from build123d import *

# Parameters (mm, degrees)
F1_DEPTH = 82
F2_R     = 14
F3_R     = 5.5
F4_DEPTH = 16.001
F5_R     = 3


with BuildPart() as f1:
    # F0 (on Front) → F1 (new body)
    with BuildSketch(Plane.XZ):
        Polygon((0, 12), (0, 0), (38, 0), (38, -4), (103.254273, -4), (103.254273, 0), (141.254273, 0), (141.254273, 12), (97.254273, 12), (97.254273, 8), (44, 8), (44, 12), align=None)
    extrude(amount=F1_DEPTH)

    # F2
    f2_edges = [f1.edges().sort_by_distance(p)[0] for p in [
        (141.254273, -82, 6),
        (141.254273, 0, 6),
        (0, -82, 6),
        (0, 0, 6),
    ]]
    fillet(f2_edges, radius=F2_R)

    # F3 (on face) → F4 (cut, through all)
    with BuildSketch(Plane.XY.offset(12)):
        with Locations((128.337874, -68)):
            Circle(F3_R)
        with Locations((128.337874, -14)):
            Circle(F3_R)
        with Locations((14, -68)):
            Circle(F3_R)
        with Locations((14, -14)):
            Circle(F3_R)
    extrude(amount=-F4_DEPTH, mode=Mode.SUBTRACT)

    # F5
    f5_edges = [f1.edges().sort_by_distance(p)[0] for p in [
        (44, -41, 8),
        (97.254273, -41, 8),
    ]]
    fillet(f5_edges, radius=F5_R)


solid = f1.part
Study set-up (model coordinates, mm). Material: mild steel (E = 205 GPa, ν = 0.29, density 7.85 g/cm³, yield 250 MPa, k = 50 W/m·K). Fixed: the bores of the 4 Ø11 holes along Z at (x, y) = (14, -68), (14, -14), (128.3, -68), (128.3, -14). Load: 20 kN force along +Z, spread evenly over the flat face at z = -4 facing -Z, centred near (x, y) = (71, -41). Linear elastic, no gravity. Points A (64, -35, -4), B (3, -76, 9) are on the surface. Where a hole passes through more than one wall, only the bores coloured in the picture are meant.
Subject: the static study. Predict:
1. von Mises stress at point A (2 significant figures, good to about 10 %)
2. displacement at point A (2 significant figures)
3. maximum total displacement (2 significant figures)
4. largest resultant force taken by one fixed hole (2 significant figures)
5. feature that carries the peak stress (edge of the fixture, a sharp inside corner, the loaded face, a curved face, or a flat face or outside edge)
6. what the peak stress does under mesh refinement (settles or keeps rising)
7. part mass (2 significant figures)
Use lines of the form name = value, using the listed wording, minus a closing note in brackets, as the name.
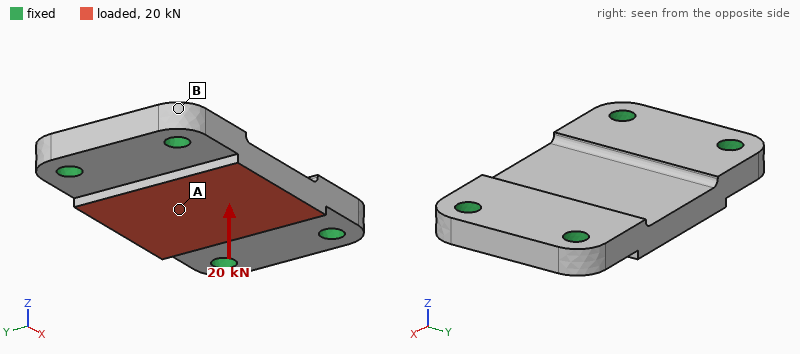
von Mises stress at point A = 62 MPa
displacement at point A = 42 µm
maximum total displacement = 45 µm
largest resultant force taken by one fixed hole = 8.3 kN
feature that carries the peak stress = edge of the fixture
what the peak stress does under mesh refinement = keeps rising
part mass = 1.1 kg
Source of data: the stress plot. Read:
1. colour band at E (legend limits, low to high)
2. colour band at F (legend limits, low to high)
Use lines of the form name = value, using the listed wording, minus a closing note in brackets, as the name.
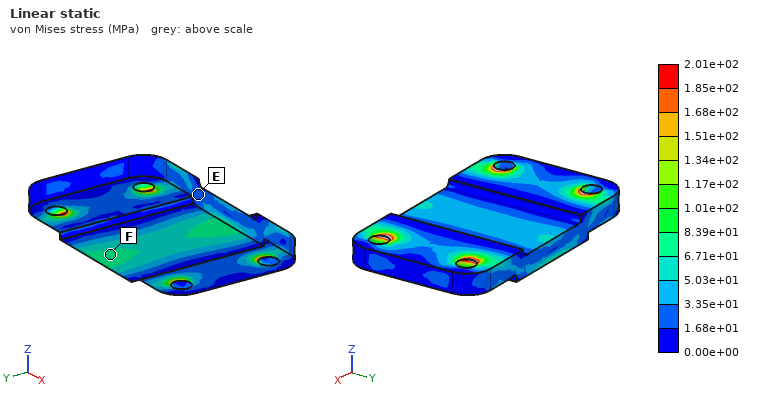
colour band at E = 1.68e+01 to 3.35e+01 MPa
colour band at F = 6.71e+01 to 8.39e+01 MPa
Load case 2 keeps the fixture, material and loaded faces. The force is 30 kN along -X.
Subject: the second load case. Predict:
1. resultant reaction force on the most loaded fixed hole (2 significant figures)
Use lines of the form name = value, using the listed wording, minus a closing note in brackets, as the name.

resultant reaction force on the most loaded fixed hole = 7.8 kN
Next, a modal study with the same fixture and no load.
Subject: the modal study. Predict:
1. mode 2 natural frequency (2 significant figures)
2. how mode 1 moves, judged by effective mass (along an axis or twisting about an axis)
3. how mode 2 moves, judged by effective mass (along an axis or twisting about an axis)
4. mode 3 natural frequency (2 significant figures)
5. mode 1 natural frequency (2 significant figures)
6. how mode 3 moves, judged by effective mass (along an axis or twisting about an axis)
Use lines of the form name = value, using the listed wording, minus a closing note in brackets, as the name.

mode 2 natural frequency = 6600 Hz
how mode 1 moves, judged by effective mass = along Z
how mode 2 moves, judged by effective mass = twisting about X
mode 3 natural frequency = 11 kHz
mode 1 natural frequency = 4900 Hz
how mode 3 moves, judged by effective mass = twisting about Y
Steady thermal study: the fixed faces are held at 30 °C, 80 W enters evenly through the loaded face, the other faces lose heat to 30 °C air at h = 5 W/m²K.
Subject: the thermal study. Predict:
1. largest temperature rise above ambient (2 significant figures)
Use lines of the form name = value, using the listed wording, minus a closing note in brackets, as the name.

largest temperature rise above ambient = 35 K
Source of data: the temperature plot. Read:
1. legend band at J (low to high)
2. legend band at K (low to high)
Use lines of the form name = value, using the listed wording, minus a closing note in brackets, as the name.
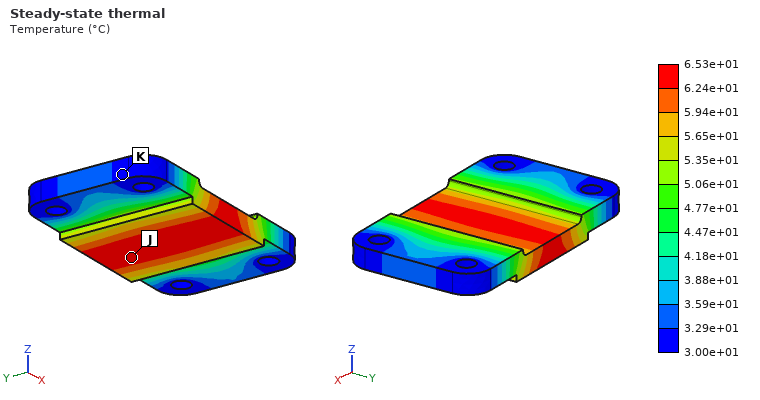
legend band at J = 6.24e+01 to 6.53e+01 °C
legend band at K = 3.00e+01 to 3.29e+01 °C
